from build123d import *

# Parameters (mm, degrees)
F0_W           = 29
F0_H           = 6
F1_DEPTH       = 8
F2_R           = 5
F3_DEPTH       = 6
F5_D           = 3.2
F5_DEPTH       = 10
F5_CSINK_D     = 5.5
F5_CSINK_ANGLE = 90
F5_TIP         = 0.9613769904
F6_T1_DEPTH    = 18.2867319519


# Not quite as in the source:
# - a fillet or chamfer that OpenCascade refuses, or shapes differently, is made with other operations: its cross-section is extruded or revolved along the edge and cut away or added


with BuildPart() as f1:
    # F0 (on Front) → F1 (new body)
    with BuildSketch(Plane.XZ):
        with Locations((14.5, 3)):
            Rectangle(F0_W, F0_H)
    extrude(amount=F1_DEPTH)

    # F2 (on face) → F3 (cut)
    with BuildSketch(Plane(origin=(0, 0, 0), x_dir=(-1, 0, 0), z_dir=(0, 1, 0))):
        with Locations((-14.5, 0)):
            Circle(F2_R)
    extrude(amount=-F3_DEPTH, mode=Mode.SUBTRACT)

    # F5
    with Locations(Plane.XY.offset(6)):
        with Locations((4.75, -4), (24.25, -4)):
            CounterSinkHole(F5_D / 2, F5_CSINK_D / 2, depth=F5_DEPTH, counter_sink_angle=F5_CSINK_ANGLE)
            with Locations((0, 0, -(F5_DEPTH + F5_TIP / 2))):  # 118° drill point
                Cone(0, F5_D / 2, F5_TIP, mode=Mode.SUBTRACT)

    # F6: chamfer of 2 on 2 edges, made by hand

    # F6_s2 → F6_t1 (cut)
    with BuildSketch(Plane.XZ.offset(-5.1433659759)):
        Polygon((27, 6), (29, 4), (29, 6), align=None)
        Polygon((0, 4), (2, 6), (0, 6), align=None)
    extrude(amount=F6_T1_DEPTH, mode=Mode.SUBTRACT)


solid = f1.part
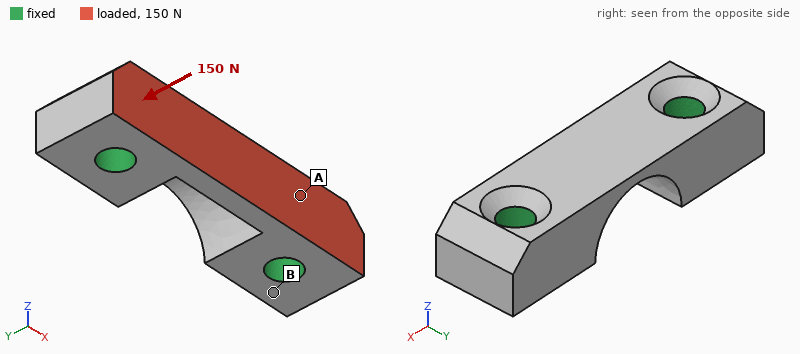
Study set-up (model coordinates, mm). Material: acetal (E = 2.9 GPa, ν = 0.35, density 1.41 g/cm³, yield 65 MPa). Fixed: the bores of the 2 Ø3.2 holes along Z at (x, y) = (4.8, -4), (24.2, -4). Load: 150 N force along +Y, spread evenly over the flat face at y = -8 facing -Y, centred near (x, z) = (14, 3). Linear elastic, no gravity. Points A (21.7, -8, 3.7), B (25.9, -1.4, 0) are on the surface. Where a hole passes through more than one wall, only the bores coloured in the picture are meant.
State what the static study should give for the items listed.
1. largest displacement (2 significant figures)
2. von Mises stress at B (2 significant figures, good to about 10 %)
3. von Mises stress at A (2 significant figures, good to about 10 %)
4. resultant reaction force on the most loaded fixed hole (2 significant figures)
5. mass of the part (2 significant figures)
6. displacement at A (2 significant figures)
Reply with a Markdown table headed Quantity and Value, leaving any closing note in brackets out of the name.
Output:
| Quantity | Value |
|---|---|
| largest displacement | 29 µm |
| von Mises stress at B | 0.85 MPa |
| von Mises stress at A | 1.9 MPa |
| resultant reaction force on the most loaded fixed hole | 77 N |
| mass of the part | 1.4 g |
| displacement at A | 4.9 µm |
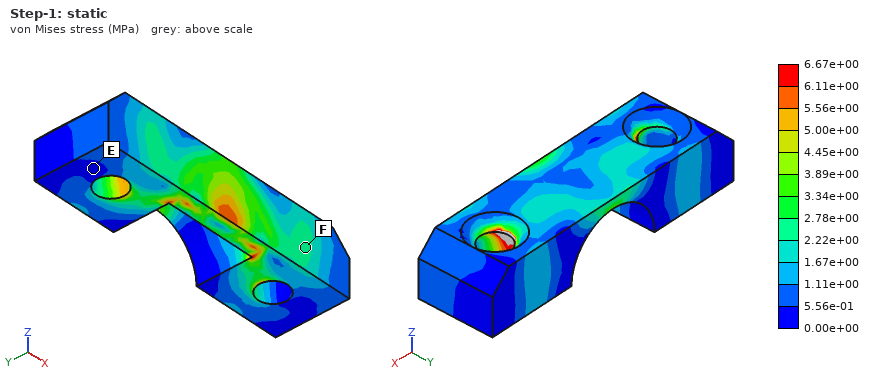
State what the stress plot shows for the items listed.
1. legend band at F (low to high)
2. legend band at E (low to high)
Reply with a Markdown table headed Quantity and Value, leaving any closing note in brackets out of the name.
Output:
| Quantity | Value |
|---|---|
| legend band at F | 2.22e+00 to 2.78e+00 MPa |
| legend band at E | 0.00e+00 to 5.56e-01 MPa |
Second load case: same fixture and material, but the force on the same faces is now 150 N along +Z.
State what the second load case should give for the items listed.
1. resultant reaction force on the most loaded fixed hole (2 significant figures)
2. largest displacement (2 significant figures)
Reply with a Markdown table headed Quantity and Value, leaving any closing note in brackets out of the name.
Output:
| Quantity | Value |
|---|---|
| resultant reaction force on the most loaded fixed hole | 76 N |
| largest displacement | 38 µm |
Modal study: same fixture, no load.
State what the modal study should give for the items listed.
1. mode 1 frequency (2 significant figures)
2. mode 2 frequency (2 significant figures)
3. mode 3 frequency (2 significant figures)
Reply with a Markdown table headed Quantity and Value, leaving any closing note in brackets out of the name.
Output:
| Quantity | Value |
|---|---|
| mode 1 frequency | 18 kHz |
| mode 2 frequency | 19 kHz |
| mode 3 frequency | 23 kHz |
